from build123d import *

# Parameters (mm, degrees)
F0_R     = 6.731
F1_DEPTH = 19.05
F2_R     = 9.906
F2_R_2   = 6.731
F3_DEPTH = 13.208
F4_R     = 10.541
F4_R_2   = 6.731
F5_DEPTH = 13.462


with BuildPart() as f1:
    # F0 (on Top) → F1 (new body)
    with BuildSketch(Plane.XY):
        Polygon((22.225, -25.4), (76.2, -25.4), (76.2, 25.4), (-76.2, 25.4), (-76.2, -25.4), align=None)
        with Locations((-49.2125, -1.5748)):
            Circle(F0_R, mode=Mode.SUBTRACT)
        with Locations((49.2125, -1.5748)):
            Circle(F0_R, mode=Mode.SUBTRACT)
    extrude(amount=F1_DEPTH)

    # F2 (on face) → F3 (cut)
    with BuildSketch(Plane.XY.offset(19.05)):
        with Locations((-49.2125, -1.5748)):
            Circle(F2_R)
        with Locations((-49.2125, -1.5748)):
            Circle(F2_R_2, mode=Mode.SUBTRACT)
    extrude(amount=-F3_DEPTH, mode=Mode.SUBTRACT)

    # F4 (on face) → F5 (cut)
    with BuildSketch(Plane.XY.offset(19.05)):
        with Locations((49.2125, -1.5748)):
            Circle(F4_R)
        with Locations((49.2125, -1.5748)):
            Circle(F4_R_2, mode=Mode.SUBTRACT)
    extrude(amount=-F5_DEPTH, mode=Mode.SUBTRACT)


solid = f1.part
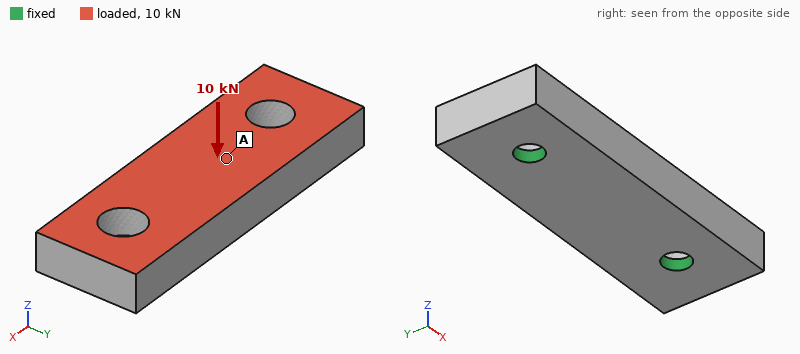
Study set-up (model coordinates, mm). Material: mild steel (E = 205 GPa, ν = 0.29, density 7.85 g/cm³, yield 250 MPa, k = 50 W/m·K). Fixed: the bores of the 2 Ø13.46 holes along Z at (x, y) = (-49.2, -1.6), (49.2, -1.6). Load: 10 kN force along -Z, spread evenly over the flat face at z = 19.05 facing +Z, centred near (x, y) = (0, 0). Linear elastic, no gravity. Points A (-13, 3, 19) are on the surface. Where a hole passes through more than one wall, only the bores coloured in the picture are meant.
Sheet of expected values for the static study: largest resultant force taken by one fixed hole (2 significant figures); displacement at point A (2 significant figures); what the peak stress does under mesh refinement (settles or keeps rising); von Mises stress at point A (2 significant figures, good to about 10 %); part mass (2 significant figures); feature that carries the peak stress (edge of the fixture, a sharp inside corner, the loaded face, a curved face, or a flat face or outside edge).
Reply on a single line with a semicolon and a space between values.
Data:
5.4 kN; 6.8 µm; keeps rising; 12 MPa; 1.1 kg; edge of the fixture
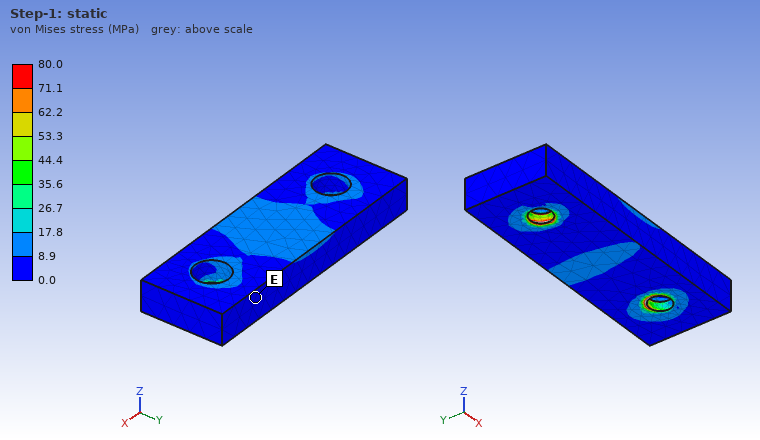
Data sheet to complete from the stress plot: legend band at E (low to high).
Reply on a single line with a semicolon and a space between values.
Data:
0.0 to 8.9 MPa
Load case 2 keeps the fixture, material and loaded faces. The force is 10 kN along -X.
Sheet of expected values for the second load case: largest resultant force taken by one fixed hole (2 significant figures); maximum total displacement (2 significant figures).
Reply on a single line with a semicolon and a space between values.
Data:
5.3 kN; 6.1 µm
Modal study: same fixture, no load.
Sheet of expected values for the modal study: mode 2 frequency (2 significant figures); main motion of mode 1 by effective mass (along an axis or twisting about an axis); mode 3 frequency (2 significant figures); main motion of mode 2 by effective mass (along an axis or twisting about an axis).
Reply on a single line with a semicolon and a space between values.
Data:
5900 Hz; along Y; 7500 Hz; along Z
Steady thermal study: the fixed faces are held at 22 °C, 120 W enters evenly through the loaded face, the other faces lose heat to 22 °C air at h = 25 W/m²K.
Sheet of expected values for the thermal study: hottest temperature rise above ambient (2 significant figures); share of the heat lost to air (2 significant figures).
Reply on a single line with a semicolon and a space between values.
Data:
41 K; 9.8 %
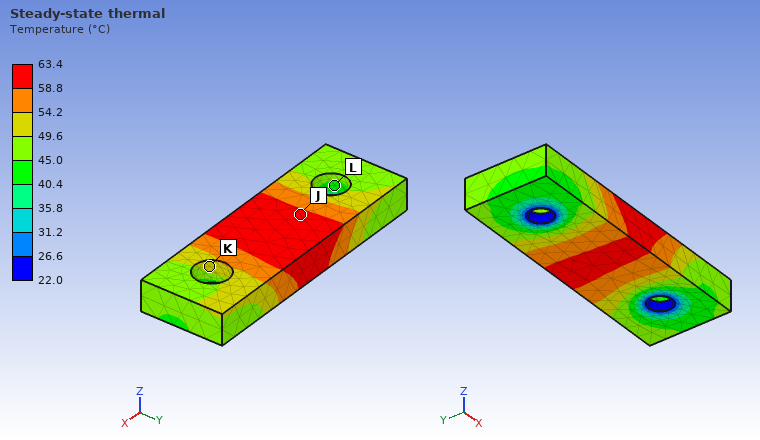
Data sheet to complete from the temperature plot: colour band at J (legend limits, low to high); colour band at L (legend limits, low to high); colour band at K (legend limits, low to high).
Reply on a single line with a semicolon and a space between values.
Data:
58.8 to 63.4 °C; 40.4 to 45.0 °C; 49.6 to 54.2 °C
